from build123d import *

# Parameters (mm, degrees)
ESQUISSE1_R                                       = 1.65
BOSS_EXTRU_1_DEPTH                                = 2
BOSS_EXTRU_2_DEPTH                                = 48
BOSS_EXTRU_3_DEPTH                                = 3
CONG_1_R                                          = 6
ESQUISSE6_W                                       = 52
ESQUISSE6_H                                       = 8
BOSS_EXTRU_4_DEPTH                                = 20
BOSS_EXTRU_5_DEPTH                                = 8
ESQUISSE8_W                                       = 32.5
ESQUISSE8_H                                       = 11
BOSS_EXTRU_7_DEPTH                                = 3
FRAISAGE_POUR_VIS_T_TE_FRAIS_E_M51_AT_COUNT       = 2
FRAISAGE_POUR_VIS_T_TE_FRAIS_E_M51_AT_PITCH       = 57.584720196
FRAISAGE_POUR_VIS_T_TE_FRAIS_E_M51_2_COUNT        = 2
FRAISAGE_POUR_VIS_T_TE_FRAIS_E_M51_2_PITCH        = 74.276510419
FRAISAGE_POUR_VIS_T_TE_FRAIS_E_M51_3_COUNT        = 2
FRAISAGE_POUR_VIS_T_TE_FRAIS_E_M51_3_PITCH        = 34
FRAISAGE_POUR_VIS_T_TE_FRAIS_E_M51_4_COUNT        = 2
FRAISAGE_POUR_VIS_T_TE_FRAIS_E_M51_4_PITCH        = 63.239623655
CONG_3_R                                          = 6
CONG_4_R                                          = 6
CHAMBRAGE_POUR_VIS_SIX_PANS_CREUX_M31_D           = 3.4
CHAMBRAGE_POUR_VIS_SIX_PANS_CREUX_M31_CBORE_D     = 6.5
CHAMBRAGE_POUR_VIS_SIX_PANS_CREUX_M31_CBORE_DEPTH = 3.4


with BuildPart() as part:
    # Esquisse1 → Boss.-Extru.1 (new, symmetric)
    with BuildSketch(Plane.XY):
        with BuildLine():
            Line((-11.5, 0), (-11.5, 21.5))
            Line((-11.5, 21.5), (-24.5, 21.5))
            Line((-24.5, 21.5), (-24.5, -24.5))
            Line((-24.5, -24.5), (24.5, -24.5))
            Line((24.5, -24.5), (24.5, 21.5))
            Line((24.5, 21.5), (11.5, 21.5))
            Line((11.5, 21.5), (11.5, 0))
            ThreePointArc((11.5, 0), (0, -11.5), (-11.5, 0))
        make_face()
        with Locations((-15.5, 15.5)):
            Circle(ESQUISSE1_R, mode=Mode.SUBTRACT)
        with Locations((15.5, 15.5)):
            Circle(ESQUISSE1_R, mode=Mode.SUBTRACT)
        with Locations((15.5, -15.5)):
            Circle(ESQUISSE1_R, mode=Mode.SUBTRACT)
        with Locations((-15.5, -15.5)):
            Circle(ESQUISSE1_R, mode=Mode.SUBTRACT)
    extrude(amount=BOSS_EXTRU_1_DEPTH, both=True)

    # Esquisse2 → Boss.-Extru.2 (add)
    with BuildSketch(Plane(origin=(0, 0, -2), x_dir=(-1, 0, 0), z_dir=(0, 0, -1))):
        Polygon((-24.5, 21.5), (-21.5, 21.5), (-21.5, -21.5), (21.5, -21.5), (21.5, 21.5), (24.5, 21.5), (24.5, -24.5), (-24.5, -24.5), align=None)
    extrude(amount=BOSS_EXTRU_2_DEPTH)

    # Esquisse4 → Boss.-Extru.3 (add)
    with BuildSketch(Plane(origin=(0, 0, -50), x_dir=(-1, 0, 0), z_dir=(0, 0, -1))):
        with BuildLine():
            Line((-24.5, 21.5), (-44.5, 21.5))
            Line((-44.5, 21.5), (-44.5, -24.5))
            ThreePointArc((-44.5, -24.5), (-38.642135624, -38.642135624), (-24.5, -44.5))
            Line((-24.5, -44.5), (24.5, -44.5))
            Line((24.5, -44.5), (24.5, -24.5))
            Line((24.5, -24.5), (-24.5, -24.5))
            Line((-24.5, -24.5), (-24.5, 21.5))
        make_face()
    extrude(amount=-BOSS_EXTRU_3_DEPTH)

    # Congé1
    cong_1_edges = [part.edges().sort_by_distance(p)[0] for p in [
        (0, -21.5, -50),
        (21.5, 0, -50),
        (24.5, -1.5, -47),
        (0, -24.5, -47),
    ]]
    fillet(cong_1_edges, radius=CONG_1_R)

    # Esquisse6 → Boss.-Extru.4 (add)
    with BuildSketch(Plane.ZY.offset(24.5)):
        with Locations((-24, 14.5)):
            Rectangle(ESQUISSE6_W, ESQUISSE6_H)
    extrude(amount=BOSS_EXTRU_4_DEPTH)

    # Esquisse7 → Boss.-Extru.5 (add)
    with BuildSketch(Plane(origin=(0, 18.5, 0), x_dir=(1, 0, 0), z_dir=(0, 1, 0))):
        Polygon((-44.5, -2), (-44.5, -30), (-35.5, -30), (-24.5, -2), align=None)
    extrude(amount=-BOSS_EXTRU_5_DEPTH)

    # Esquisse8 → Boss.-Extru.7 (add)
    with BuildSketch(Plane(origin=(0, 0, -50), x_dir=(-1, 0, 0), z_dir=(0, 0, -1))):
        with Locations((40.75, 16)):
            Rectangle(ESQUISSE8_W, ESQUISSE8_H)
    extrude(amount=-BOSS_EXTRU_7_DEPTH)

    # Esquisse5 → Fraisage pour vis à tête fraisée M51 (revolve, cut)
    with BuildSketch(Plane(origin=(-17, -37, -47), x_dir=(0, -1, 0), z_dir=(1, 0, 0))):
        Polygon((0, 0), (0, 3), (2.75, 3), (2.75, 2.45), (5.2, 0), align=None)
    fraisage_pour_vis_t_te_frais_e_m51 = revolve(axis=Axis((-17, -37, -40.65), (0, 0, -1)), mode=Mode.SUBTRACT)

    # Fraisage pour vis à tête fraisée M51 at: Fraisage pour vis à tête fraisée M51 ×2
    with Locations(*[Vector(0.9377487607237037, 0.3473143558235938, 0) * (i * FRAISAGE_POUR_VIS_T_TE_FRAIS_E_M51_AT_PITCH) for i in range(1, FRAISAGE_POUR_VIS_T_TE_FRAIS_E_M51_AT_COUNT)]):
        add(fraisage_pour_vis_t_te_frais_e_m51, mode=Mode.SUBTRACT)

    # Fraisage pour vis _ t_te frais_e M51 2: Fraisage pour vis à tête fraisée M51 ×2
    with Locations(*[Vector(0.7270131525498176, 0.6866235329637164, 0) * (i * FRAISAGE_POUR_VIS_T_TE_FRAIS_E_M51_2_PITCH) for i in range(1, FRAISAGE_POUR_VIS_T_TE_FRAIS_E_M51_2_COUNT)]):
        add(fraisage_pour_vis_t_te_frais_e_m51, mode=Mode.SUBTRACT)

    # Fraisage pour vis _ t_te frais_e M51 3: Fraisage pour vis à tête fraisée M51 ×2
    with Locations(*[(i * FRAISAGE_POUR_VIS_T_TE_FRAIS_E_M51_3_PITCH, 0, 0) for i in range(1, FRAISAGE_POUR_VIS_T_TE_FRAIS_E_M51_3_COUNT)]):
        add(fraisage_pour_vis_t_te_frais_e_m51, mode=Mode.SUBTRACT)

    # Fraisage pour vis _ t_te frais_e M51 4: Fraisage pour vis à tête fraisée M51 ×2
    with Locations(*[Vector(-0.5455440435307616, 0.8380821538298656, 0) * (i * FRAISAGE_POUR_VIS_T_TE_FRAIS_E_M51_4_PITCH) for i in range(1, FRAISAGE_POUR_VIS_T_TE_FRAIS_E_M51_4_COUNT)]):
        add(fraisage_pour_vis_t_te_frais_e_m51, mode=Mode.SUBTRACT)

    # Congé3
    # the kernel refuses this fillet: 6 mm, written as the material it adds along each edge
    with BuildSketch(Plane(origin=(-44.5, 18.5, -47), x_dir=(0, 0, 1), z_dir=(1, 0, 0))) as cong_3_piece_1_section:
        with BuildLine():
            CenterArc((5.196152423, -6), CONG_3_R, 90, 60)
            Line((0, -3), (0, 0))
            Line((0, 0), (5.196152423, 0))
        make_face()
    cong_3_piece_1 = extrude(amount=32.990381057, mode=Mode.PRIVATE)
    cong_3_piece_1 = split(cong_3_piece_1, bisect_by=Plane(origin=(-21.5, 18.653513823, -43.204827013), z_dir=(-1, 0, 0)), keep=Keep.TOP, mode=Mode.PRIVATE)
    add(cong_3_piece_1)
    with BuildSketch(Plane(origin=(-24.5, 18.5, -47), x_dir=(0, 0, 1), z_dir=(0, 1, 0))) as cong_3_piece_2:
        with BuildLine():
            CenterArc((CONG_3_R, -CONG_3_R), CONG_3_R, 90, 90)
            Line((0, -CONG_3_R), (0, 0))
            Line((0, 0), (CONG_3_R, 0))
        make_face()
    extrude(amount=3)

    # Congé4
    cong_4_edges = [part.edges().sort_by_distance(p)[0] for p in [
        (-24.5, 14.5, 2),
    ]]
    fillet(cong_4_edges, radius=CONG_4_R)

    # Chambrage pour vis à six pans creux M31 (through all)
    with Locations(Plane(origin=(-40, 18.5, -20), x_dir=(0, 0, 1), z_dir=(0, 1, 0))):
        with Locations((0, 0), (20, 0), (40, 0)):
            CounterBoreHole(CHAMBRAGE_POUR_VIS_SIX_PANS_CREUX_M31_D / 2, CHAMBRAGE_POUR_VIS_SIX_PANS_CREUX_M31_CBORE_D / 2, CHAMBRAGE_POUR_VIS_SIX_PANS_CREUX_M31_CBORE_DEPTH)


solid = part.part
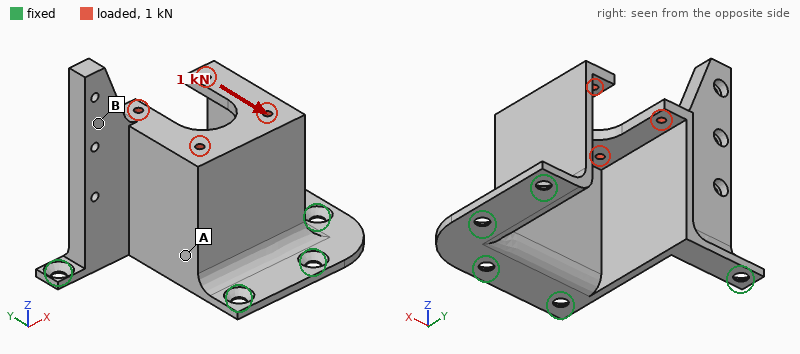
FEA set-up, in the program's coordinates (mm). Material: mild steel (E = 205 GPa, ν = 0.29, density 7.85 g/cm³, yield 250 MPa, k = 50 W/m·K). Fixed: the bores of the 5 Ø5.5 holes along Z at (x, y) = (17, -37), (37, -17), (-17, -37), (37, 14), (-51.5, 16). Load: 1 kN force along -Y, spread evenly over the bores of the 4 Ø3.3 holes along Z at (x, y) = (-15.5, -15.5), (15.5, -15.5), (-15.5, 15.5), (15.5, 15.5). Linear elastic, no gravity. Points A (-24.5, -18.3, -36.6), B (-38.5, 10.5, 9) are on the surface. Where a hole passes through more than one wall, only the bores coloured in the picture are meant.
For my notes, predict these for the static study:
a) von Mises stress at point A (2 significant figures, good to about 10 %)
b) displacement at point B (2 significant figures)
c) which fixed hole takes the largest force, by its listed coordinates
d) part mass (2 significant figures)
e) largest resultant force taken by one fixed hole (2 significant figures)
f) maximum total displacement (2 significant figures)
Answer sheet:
24 MPa
0.086 mm
(-17, -37)
340 g
970 N
0.12 mm
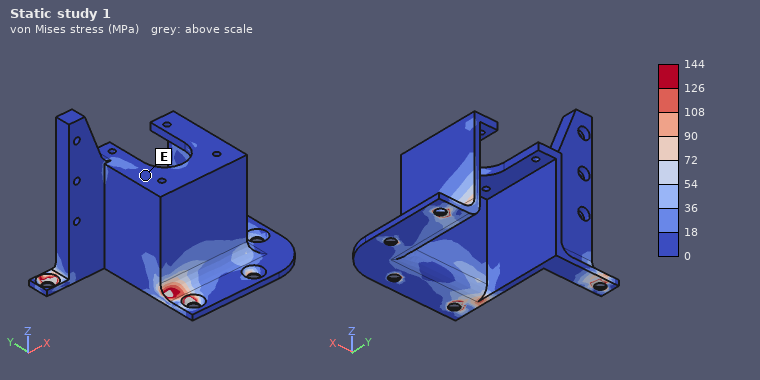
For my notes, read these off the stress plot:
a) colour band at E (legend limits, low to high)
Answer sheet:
0 to 18 MPa
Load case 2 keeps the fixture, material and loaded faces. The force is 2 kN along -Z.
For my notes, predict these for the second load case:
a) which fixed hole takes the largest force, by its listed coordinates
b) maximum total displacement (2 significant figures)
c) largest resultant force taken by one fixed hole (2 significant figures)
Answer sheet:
(-51.5, 16)
0.11 mm
900 N
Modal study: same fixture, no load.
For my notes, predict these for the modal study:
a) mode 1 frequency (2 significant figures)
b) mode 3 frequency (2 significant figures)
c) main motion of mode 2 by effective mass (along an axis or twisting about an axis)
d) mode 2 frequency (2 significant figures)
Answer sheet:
830 Hz
3000 Hz
along Y
2000 Hz
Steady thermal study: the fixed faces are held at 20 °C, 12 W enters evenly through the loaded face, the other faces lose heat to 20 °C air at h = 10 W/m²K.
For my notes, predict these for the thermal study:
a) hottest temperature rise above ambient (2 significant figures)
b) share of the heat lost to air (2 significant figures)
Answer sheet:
41 K
35 %
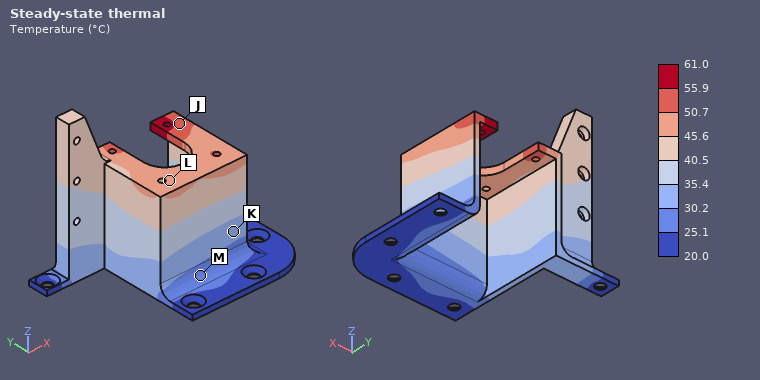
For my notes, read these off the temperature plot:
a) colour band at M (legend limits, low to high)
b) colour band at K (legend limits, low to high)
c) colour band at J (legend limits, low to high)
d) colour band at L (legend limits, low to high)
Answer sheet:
25.1 to 30.2 °C
30.2 to 35.4 °C
50.7 to 55.9 °C
45.6 to 50.7 °C
